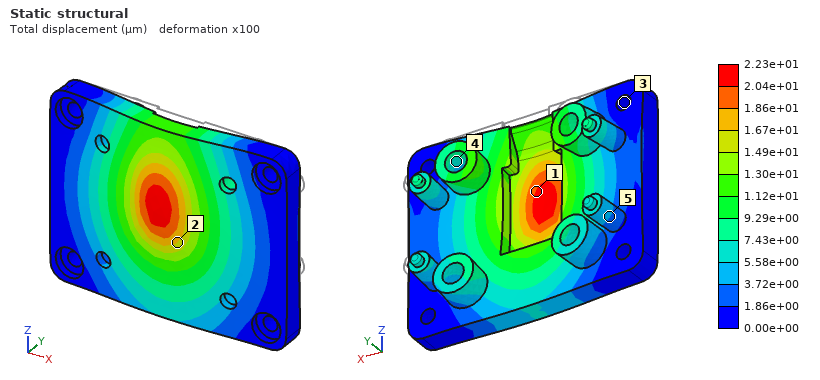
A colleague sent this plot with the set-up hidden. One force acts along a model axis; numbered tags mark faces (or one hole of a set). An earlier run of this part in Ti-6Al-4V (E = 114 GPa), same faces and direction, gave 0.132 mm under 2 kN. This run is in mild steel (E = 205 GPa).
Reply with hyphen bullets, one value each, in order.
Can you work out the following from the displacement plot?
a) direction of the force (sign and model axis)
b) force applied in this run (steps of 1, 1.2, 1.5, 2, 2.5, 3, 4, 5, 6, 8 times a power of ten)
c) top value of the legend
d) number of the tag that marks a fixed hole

- -Y
- 600 N
- 2.23e+01 µm
- 3
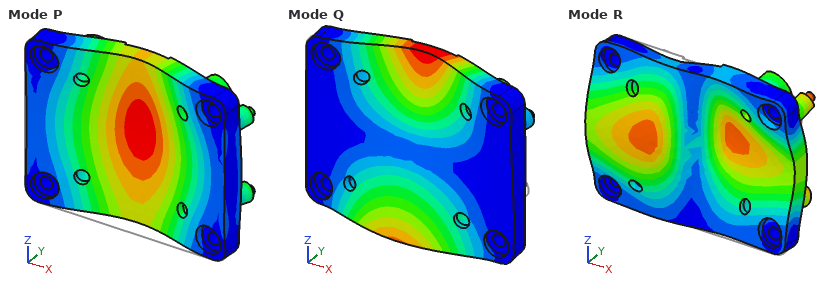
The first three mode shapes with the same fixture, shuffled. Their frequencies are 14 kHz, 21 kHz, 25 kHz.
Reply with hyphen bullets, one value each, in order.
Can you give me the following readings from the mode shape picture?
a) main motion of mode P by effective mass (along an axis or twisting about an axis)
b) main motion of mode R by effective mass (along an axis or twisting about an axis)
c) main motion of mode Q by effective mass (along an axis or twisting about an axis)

- along Y
- twisting about Z
- twisting about X
